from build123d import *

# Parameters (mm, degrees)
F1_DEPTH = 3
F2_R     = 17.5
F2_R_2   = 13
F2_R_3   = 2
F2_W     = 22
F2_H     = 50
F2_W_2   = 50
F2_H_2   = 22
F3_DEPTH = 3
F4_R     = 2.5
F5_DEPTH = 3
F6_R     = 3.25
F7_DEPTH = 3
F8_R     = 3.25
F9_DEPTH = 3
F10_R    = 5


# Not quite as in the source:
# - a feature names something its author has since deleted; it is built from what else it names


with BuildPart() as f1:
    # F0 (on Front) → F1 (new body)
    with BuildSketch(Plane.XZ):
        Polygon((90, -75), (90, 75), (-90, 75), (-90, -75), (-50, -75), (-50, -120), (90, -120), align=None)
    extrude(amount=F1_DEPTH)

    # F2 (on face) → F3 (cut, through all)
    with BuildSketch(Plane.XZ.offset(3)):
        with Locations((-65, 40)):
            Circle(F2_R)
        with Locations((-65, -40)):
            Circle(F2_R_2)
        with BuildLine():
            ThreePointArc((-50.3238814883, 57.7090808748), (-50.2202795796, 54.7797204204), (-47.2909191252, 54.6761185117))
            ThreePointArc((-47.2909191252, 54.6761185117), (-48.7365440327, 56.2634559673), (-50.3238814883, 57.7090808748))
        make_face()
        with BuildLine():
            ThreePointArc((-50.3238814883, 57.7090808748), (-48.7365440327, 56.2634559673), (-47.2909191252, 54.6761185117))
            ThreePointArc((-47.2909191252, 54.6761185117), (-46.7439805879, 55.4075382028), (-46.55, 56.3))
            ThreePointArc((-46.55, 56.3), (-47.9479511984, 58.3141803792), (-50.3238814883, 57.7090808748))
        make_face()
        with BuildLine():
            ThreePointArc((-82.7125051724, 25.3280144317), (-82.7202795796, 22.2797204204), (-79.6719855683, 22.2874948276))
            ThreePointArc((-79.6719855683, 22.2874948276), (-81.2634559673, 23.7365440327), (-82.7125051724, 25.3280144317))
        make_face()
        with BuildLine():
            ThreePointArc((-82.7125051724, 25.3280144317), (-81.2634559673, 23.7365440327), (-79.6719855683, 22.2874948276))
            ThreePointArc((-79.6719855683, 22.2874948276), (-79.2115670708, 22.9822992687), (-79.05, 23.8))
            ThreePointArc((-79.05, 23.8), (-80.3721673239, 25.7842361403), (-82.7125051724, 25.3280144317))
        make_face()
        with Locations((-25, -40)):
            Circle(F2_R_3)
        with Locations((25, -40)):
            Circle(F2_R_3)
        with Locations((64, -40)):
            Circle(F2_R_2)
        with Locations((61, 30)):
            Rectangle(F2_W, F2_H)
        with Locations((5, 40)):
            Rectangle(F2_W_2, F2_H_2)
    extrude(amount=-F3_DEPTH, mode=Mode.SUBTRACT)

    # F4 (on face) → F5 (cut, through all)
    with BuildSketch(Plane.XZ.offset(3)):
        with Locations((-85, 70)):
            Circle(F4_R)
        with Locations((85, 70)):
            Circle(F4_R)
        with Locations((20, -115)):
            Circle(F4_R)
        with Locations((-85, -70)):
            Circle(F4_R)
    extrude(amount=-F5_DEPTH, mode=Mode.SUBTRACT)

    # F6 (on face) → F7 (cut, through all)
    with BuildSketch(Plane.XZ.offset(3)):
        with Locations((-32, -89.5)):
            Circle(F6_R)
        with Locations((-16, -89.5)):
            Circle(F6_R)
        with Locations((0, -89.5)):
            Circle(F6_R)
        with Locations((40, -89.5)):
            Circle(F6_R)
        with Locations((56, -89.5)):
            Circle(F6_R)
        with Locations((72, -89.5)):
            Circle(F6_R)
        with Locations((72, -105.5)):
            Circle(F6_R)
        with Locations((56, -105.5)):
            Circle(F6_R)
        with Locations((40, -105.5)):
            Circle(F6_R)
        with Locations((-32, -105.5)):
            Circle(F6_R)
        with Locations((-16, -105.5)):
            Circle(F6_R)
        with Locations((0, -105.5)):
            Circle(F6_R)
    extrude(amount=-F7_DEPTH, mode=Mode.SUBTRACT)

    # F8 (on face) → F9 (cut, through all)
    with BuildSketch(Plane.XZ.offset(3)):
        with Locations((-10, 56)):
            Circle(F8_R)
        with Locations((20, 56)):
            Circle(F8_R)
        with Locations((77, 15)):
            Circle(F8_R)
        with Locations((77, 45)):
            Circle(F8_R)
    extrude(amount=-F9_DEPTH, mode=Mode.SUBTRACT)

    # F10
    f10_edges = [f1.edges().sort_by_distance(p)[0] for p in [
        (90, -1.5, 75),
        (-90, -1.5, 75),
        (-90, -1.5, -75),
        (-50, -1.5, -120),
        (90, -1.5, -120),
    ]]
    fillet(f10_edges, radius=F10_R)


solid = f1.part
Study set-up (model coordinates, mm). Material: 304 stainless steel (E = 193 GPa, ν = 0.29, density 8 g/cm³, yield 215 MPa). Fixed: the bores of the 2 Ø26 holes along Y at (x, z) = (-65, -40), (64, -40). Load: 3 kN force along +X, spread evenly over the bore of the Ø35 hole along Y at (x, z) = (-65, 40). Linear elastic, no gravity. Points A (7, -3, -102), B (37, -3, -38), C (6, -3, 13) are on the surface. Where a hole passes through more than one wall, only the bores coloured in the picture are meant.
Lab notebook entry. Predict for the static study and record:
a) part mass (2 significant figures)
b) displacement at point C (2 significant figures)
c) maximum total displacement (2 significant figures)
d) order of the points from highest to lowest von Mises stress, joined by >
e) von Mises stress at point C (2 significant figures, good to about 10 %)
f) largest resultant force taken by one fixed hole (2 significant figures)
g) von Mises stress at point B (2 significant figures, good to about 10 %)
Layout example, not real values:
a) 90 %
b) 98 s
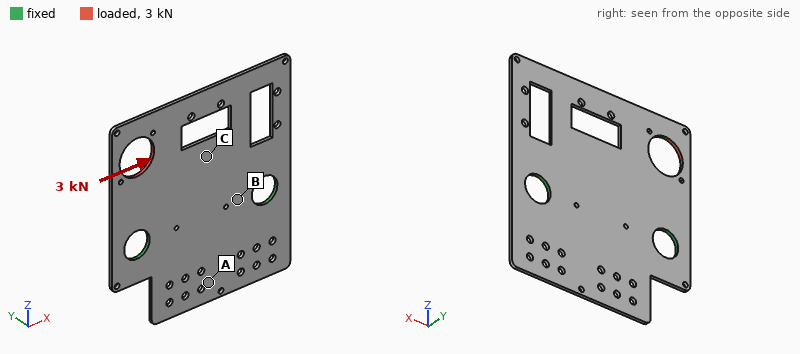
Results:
a) 680 g
b) 5.1 µm
c) 28 µm
d) C > B > A
e) 15 MPa
f) 2.3 kN
g) 8.6 MPa
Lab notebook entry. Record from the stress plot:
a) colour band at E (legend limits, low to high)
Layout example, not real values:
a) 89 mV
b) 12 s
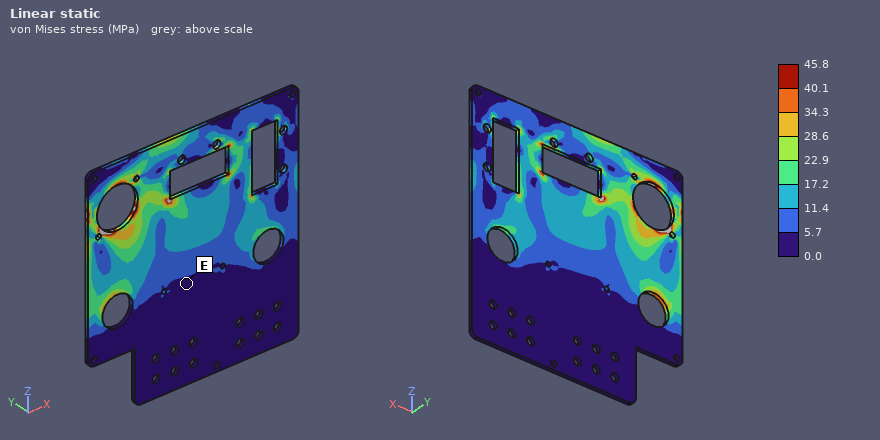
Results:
a) 0.0 to 5.7 MPa
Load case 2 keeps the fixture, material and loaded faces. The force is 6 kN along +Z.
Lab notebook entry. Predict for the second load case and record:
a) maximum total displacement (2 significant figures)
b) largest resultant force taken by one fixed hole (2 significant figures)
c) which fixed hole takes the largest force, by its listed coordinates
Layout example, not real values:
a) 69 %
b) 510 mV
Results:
a) 31 µm
b) 5.9 kN
c) (-65, -40)
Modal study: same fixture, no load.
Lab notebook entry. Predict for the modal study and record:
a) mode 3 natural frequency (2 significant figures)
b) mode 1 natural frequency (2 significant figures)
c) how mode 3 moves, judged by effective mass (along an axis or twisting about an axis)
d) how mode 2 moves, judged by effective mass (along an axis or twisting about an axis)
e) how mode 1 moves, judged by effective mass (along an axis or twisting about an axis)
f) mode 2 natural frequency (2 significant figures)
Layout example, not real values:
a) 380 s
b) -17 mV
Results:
a) 430 Hz
b) 210 Hz
c) along Y
d) twisting about Z
e) along Y
f) 380 Hz
